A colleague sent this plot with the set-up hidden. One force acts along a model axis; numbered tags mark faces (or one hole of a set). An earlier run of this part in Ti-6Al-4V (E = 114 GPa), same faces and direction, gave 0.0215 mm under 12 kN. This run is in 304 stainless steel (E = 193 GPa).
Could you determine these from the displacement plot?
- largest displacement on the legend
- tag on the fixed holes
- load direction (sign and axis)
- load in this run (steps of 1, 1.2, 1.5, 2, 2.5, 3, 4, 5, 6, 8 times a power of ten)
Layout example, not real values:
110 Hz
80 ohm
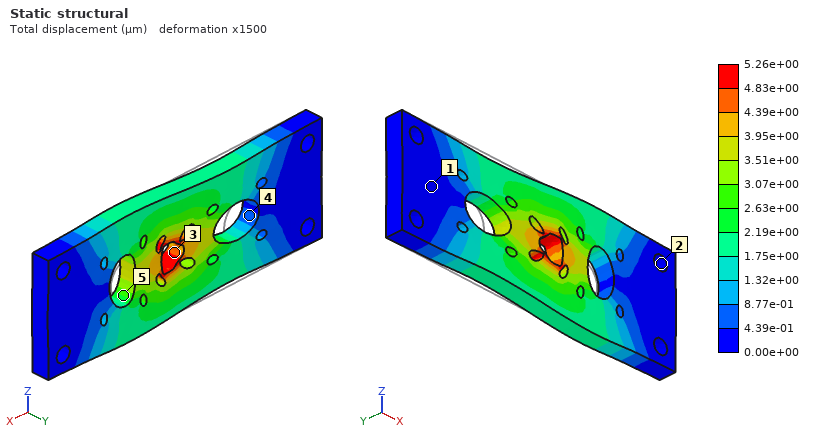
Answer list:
5.26e+00 µm
2
+X
5 kN
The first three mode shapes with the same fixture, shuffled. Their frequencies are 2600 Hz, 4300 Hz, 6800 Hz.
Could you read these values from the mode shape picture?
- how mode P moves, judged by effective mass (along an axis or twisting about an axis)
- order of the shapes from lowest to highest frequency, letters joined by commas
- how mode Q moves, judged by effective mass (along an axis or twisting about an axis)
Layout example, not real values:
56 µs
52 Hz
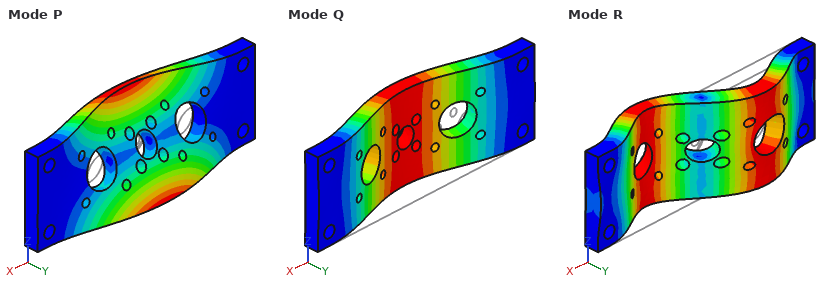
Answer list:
twisting about X
Q, P, R
along Y
